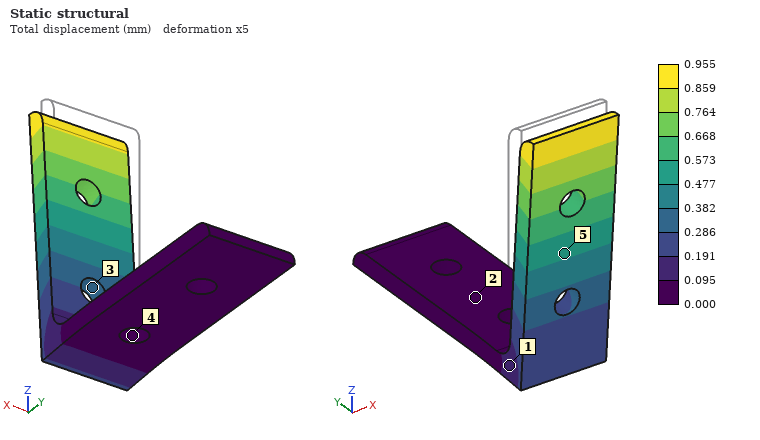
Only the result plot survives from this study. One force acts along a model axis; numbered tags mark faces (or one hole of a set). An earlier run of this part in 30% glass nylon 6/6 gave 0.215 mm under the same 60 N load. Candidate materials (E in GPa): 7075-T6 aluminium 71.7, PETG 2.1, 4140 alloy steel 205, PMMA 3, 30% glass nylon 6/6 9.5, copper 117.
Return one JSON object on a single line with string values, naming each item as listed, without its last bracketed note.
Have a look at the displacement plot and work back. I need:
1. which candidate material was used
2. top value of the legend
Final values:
{"which candidate material was used": "PETG", "top value of the legend": "0.955 mm"}
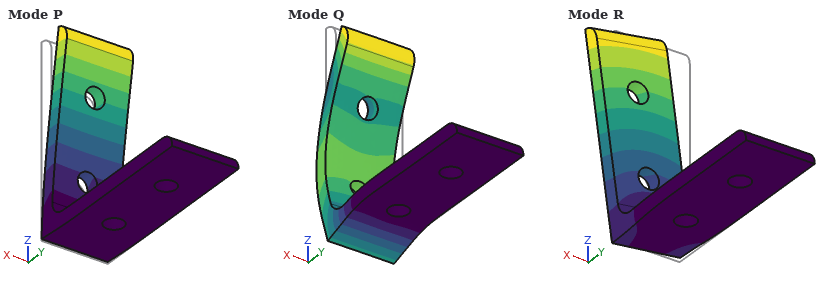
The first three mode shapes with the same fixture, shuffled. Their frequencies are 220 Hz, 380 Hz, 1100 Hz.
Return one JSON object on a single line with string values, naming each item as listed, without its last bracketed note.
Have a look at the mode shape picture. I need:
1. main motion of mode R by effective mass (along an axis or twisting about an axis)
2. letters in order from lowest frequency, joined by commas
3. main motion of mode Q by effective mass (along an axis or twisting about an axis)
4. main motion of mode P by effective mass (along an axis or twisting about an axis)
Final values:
{"main motion of mode R by effective mass": "along X", "letters in order from lowest frequency, joined by commas": "P, R, Q", "main motion of mode Q by effective mass": "along Z", "main motion of mode P by effective mass": "along Y"}
